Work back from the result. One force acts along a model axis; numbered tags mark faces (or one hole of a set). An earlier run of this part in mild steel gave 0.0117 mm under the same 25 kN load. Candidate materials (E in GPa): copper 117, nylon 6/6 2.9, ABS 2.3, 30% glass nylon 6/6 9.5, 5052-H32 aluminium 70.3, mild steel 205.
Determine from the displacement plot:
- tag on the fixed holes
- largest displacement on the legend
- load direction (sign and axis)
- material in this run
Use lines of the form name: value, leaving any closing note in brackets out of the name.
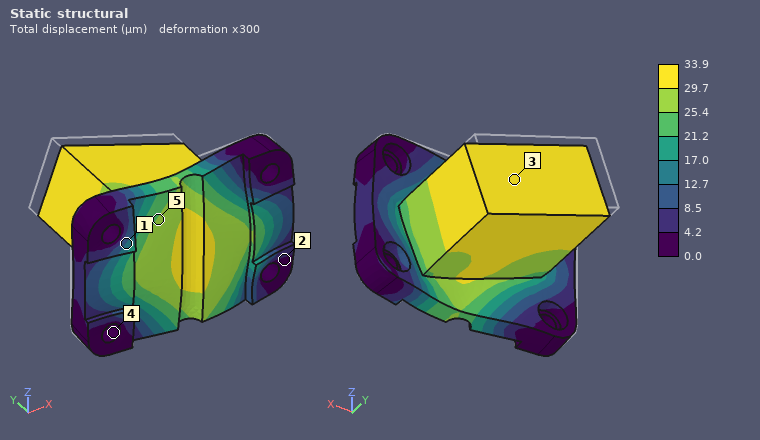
tag on the fixed holes: 4
largest displacement on the legend: 33.9 µm
load direction: -Y
material in this run: 5052-H32 aluminium
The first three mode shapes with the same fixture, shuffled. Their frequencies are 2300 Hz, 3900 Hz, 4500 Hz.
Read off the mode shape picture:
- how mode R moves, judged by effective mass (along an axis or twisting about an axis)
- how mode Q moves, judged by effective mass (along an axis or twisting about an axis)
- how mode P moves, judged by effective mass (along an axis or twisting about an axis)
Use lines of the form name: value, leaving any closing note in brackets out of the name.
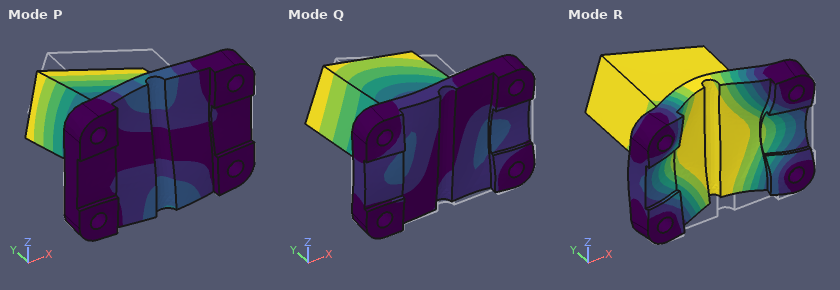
how mode R moves, judged by effective mass: along Y
how mode Q moves, judged by effective mass: along X
how mode P moves, judged by effective mass: along Z
